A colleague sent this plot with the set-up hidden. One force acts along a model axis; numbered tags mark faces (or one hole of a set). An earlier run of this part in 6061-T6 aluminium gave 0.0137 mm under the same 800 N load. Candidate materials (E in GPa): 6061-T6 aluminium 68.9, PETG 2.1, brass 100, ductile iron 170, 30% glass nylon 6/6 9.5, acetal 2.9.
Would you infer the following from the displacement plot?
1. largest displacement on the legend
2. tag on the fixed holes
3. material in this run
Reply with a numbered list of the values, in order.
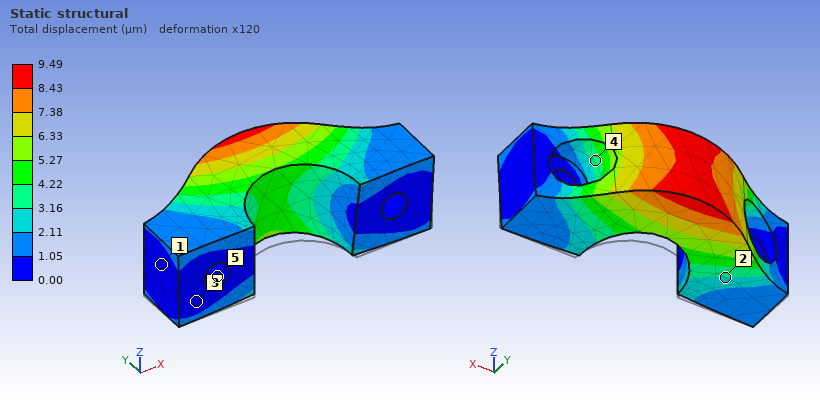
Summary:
1. 9.49 µm
2. 5
3. brass
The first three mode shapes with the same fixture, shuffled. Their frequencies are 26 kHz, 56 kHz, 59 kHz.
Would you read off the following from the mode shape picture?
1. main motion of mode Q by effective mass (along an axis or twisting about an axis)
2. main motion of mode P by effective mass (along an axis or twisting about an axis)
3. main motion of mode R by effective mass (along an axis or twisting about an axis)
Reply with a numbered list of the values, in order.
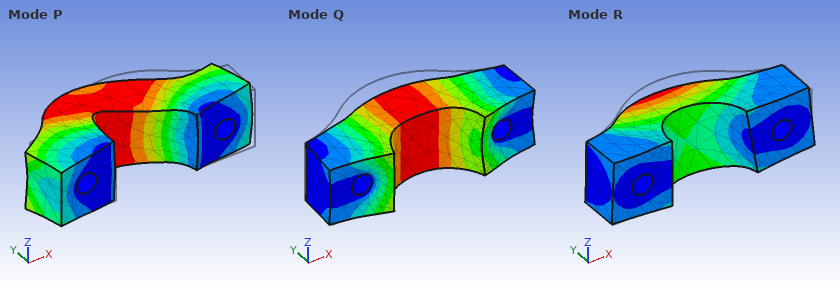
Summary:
1. along Y
2. along X
3. along Z
